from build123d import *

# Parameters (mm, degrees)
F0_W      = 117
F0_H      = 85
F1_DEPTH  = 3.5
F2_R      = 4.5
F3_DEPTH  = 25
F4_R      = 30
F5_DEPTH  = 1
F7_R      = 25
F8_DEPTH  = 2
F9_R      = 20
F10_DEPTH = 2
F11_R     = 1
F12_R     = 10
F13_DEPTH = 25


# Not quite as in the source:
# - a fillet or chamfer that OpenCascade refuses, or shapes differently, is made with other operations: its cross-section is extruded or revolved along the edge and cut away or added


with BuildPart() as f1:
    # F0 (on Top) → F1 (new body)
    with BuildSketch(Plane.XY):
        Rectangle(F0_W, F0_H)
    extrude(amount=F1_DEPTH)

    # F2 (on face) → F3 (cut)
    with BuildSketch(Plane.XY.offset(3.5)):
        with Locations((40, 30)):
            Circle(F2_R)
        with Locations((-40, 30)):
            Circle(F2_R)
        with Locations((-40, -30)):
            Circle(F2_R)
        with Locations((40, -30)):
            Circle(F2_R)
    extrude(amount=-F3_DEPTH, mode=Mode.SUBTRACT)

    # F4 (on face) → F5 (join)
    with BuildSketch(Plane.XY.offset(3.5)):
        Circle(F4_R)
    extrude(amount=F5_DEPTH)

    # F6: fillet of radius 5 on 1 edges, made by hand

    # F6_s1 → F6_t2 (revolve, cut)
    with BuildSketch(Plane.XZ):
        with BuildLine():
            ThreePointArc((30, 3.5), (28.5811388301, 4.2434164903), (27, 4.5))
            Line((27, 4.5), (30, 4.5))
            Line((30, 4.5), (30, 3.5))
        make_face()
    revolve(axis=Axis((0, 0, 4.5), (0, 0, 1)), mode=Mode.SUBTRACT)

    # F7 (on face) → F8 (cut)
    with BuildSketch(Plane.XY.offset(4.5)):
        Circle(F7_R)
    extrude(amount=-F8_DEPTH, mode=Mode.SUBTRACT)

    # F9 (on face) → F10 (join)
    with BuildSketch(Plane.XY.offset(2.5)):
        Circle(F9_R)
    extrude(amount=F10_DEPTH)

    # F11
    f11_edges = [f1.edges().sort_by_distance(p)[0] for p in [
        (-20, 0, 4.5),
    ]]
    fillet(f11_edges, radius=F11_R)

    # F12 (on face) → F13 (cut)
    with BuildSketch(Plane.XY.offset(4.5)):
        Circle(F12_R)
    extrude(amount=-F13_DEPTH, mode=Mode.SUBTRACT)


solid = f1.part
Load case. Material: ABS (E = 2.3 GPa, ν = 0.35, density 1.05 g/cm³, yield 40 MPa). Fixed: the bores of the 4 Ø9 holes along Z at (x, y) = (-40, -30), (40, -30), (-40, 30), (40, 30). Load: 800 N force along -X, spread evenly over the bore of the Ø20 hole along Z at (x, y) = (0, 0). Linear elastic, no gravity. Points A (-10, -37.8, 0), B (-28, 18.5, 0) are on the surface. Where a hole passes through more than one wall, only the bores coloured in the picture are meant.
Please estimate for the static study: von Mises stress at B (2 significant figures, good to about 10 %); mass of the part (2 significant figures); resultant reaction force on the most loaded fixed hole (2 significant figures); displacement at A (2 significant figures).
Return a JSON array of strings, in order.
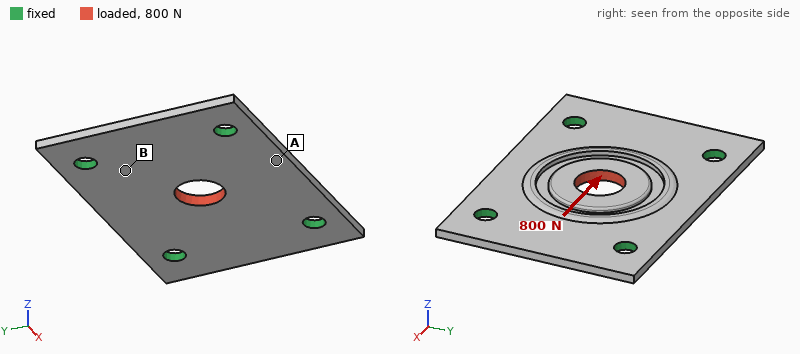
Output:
["2.8 MPa", "35 g", "210 N", "12 µm"]
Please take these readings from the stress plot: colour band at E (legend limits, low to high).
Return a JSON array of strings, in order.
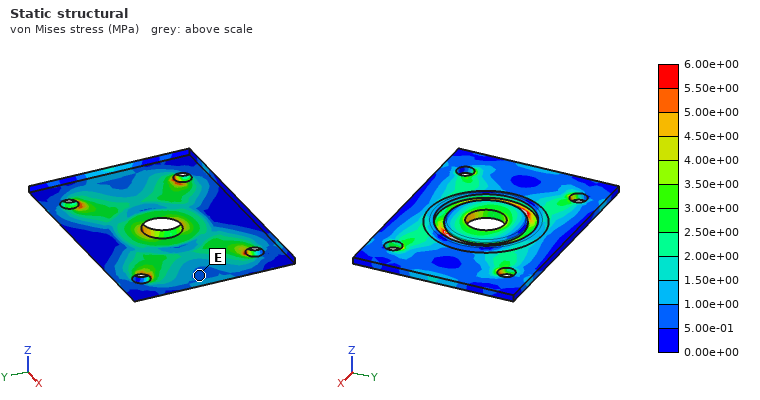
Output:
["5.00e-01 to 1.00e+00 MPa"]
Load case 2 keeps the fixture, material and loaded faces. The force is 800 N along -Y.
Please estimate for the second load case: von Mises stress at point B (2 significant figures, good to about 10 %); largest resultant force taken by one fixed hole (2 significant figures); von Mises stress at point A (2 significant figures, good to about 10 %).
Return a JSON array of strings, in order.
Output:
["3.0 MPa", "230 N", "1.9 MPa"]
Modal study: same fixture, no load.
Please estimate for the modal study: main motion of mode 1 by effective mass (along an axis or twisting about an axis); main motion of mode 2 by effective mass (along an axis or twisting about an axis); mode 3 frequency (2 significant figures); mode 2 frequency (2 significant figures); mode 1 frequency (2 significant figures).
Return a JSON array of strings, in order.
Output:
["along Z", "twisting about X", "1400 Hz", "1100 Hz", "850 Hz"]
